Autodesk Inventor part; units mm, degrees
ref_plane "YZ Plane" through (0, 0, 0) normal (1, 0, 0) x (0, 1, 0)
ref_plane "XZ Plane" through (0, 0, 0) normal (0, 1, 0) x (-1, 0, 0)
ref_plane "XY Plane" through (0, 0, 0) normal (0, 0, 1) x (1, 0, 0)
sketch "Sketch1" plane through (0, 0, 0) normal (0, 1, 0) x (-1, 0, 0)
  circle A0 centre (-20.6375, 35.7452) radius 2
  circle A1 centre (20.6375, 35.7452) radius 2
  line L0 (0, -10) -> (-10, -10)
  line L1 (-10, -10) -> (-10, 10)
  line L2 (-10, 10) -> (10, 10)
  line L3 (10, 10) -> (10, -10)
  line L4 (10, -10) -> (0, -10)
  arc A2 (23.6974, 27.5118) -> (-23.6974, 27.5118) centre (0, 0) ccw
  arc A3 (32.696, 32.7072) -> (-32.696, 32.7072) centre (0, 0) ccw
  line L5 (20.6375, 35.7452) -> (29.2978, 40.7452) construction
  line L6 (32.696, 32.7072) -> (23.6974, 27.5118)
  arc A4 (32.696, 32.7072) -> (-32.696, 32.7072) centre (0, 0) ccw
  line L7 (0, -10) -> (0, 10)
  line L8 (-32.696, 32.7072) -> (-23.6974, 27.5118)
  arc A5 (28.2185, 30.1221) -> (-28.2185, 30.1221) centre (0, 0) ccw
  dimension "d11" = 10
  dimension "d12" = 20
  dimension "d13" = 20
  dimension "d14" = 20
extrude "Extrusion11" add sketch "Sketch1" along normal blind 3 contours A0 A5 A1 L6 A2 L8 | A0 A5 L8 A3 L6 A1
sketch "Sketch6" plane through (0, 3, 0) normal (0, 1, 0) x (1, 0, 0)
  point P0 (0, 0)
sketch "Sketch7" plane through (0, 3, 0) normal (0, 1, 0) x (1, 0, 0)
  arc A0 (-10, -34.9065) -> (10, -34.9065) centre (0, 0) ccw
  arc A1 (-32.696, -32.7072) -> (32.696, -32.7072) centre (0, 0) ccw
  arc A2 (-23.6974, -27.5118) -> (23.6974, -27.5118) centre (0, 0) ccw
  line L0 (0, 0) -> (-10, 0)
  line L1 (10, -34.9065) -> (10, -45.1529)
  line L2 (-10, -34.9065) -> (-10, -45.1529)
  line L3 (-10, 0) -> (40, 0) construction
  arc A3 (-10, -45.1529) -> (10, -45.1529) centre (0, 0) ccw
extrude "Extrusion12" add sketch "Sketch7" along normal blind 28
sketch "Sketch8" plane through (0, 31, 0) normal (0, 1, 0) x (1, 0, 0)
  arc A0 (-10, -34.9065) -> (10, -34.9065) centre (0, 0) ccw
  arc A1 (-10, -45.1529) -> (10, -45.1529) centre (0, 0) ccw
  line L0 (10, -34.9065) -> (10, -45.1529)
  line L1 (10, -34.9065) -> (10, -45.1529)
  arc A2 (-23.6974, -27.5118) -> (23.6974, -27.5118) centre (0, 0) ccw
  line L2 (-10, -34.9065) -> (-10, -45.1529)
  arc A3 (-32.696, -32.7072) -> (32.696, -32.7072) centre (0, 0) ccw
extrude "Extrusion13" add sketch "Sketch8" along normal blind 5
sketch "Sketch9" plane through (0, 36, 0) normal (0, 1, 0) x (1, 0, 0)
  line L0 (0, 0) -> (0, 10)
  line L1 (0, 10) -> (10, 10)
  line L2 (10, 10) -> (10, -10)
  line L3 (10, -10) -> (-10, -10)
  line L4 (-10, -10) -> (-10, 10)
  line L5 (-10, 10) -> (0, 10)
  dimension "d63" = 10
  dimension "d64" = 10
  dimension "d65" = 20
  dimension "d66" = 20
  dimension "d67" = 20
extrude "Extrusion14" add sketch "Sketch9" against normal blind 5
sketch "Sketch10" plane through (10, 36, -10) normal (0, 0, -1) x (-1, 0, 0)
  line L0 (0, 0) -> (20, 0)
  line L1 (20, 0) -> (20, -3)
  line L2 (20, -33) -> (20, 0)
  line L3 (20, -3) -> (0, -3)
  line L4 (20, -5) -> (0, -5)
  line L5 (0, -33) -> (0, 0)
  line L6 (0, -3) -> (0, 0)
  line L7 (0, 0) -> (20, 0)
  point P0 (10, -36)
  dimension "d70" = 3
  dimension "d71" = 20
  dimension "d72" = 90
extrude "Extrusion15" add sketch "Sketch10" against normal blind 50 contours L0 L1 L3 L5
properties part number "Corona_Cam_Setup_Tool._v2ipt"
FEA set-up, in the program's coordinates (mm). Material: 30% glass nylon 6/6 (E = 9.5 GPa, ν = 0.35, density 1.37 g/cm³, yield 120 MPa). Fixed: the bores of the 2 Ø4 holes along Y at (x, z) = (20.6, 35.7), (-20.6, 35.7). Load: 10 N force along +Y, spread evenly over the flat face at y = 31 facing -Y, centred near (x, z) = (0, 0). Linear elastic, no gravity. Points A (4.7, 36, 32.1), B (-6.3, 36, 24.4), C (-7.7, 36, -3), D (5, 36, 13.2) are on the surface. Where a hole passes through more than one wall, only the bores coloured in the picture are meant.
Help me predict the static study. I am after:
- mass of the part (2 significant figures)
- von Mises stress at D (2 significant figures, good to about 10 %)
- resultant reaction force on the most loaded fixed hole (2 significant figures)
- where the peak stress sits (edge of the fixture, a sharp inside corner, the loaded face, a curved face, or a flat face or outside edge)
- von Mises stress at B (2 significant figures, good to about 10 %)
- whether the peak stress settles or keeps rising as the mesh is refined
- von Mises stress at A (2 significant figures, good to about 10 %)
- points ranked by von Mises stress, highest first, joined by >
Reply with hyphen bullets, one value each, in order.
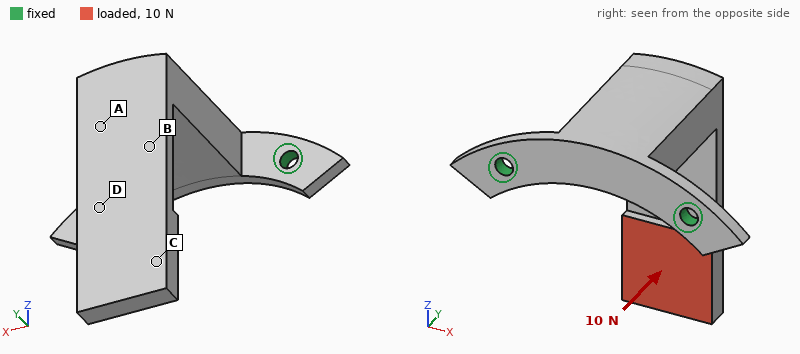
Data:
- 16 g
- 4.3 MPa
- 7.2 N
- edge of the fixture
- 8.0 MPa
- keeps rising
- 9.9 MPa
- A > B > D > C
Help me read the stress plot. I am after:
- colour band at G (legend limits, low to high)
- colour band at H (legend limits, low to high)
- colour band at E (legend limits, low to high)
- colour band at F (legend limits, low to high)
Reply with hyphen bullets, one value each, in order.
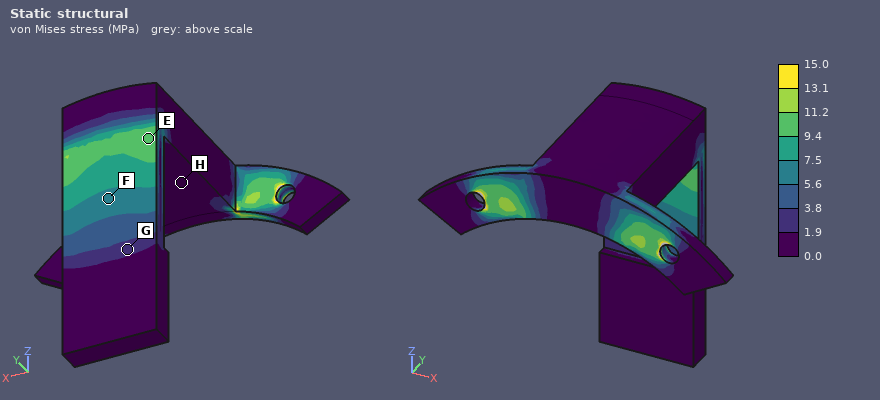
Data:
- 1.9 to 3.8 MPa
- 0.0 to 1.9 MPa
- 9.4 to 11.2 MPa
- 5.6 to 7.5 MPa
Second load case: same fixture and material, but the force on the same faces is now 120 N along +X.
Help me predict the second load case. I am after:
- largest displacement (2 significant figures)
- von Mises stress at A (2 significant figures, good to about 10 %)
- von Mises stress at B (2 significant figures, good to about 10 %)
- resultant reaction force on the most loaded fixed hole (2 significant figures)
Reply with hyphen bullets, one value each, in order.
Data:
- 1.1 mm
- 13 MPa
- 13 MPa
- 190 N
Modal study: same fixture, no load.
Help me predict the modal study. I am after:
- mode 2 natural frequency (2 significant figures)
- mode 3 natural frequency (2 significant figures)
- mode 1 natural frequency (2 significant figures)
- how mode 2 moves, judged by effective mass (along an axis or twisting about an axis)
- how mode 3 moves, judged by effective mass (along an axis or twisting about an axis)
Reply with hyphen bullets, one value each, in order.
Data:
- 600 Hz
- 920 Hz
- 280 Hz
- along Z
- along X
